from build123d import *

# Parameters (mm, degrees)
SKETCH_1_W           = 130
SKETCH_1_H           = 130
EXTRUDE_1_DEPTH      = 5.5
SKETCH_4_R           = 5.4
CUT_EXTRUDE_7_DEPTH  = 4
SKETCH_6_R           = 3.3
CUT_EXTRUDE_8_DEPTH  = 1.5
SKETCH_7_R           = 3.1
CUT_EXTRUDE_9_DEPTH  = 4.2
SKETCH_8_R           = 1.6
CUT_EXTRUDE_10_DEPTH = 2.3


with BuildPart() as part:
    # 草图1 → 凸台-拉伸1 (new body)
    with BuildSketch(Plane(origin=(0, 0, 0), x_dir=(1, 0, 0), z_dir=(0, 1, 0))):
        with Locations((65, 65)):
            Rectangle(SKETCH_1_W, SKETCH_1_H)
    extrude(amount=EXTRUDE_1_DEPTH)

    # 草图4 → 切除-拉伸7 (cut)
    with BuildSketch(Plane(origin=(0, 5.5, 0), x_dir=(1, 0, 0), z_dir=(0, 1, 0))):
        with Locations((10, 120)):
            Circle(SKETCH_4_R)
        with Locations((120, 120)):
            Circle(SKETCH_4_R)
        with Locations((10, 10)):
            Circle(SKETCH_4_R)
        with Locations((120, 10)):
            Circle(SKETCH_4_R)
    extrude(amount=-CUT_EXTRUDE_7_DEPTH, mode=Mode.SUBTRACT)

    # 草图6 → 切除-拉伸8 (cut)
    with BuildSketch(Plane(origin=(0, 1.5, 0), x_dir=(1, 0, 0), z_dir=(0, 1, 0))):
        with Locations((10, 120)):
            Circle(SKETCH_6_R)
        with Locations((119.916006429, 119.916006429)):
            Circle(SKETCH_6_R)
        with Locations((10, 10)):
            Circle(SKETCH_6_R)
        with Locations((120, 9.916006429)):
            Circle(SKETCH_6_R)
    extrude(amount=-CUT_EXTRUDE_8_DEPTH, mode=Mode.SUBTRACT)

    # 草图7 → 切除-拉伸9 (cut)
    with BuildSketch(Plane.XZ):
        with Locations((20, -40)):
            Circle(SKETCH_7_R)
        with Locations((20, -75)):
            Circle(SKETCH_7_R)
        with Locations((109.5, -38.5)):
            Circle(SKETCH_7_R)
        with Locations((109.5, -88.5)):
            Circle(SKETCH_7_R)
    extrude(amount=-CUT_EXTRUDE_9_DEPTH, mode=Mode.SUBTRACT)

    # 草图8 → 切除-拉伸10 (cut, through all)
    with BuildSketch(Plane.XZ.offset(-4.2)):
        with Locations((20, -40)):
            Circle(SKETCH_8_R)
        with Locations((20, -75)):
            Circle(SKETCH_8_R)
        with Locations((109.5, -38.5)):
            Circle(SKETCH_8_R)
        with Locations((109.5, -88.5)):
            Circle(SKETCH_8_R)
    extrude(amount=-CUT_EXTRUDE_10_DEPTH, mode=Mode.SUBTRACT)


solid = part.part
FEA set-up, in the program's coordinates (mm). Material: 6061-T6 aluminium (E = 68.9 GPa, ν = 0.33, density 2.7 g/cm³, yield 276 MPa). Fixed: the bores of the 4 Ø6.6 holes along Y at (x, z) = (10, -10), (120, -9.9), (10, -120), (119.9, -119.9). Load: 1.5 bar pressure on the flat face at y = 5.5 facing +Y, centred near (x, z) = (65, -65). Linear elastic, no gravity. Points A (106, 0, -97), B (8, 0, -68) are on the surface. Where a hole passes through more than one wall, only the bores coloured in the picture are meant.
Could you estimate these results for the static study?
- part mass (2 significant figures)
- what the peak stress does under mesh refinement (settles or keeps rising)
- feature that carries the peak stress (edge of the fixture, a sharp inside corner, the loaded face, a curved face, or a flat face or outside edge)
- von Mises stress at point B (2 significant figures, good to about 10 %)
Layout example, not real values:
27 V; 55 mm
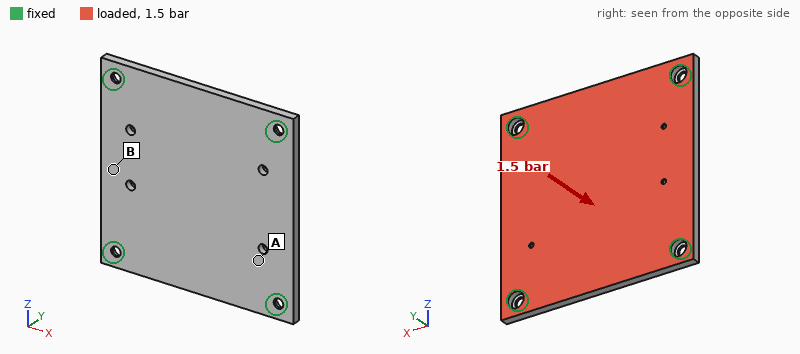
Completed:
240 g; keeps rising; edge of the fixture; 23 MPa
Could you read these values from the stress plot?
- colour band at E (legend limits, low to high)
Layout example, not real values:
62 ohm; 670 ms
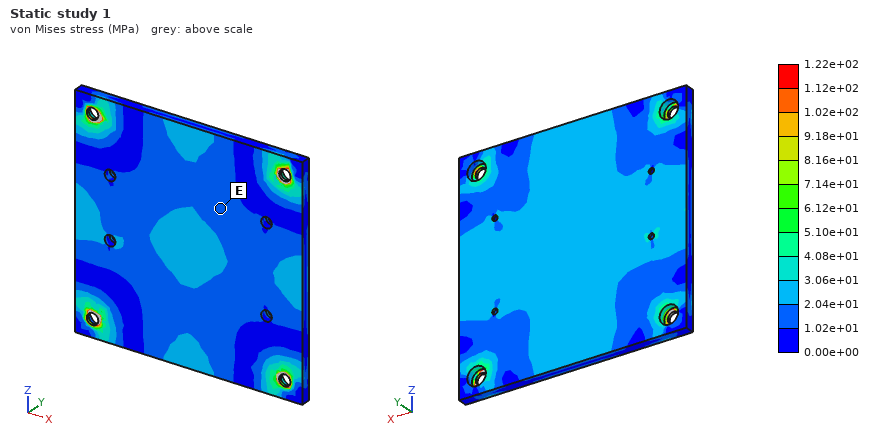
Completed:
1.02e+01 to 2.04e+01 MPa
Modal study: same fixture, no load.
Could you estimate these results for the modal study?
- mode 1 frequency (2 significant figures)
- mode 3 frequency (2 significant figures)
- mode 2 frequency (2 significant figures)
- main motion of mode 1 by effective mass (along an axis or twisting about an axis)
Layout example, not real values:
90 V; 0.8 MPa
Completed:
1300 Hz; 2200 Hz; 2200 Hz; along Y
